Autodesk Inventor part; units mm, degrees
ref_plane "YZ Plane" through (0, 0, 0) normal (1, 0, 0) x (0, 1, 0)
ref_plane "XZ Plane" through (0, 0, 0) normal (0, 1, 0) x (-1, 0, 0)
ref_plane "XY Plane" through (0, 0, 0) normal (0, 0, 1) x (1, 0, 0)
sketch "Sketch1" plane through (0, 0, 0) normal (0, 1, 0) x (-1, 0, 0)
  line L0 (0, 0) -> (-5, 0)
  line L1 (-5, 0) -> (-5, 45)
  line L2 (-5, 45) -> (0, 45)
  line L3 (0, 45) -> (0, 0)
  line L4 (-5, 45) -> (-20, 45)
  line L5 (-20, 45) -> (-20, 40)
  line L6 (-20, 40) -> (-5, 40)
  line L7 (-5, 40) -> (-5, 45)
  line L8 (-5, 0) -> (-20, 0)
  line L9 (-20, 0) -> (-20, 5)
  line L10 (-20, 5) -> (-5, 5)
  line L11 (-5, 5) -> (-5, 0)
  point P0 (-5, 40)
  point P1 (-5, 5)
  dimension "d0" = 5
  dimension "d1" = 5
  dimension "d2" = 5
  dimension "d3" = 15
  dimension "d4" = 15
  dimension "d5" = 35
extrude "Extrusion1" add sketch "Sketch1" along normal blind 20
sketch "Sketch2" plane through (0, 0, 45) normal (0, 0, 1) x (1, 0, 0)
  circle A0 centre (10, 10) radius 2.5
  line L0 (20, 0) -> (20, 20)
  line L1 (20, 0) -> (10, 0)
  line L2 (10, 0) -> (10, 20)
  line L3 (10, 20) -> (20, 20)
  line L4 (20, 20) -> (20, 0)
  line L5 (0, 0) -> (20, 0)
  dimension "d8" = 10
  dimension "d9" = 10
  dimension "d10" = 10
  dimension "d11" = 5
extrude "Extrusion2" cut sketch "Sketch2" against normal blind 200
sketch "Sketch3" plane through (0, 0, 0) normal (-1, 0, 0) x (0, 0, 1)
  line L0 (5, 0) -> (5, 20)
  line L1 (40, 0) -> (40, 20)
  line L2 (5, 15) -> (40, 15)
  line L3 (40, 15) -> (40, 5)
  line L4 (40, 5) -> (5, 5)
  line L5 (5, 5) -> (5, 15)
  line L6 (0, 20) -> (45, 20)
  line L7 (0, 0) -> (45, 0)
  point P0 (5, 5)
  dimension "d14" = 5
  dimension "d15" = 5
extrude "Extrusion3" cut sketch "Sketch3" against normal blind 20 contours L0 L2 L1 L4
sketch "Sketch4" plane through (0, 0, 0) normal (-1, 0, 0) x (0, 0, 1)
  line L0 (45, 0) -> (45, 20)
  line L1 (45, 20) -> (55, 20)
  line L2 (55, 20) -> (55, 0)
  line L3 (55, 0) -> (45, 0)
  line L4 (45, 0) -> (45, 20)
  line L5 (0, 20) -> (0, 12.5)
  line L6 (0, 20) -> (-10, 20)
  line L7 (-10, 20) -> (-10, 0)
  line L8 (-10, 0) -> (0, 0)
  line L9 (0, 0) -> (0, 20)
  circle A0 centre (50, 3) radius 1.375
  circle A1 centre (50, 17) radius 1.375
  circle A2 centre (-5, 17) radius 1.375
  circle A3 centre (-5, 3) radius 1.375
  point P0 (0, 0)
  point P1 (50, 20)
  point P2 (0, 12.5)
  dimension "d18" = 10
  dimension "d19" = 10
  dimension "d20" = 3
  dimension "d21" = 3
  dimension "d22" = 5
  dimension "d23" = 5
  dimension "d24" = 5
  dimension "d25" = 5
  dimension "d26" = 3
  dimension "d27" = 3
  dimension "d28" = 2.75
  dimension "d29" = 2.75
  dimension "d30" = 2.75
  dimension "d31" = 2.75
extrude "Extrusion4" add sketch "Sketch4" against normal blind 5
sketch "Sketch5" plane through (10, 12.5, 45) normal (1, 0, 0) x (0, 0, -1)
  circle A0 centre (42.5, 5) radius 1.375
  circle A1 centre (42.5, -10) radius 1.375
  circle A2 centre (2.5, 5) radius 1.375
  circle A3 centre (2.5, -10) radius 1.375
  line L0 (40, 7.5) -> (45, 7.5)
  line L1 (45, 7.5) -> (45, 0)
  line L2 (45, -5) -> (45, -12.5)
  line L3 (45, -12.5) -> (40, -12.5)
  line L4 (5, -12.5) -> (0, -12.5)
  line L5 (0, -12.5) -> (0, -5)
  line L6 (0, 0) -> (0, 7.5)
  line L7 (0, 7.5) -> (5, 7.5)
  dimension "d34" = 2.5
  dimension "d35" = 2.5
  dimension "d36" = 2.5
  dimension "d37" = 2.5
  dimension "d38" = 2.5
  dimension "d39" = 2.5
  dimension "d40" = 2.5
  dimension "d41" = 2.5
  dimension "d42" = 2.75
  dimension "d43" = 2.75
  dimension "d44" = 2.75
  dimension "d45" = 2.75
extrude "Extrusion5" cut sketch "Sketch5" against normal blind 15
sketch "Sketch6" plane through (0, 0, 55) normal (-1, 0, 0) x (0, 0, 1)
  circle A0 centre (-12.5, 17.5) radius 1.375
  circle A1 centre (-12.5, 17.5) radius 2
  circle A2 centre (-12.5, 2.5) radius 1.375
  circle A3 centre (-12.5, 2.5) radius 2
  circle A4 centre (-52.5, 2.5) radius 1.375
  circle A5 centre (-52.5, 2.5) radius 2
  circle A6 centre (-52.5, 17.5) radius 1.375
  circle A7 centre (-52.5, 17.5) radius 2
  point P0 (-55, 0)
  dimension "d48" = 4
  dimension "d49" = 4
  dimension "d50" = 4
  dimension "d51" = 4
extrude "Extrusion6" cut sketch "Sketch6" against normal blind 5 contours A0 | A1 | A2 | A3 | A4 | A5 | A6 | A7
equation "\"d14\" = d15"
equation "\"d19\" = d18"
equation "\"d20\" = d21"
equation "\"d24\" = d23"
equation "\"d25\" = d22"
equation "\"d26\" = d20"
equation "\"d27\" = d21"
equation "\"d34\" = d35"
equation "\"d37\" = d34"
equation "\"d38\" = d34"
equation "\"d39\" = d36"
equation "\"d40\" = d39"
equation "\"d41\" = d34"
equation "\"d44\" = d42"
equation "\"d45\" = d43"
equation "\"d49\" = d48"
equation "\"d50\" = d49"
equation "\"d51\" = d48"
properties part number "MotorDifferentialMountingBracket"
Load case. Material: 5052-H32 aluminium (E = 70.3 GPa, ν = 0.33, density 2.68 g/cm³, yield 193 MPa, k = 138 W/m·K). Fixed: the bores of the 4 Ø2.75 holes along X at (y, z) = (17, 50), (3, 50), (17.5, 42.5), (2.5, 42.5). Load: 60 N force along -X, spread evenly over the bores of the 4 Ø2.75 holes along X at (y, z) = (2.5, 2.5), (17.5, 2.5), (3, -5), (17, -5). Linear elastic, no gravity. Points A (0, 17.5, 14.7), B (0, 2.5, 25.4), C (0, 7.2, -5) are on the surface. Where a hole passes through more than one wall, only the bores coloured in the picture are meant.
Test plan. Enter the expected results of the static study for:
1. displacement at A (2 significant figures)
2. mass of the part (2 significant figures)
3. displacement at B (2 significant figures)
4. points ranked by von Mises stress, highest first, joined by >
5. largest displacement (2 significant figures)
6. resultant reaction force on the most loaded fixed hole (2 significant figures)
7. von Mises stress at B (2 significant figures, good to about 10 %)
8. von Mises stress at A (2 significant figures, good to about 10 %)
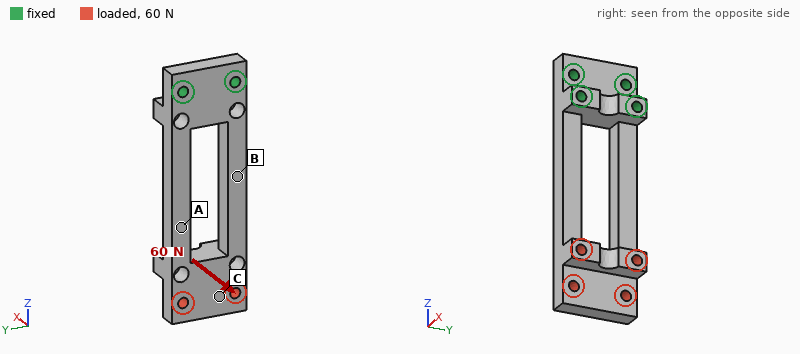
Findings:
0.13 mm
14 g
0.059 mm
B > A > C
0.34 mm
210 N
38 MPa
23 MPa
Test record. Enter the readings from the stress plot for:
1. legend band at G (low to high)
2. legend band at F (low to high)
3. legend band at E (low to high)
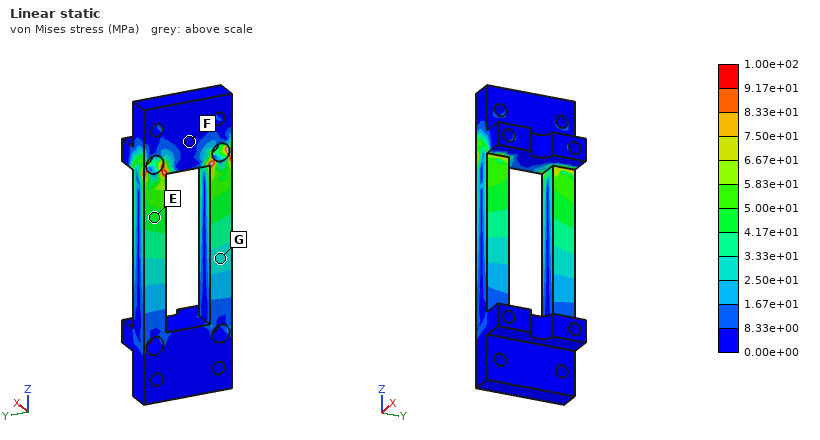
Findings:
2.50e+01 to 3.33e+01 MPa
0.00e+00 to 8.33e+00 MPa
4.17e+01 to 5.00e+01 MPa
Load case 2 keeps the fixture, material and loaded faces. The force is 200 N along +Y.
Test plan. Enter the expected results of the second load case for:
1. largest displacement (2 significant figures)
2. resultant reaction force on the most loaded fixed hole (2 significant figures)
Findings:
0.25 mm
250 N
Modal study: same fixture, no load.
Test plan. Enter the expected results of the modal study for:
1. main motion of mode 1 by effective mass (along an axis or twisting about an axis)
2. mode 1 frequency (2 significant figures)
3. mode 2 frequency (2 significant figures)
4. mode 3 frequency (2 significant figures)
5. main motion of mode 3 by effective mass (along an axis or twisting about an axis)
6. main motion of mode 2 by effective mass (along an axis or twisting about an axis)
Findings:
along X
1000 Hz
2000 Hz
4200 Hz
twisting about Z
along Y
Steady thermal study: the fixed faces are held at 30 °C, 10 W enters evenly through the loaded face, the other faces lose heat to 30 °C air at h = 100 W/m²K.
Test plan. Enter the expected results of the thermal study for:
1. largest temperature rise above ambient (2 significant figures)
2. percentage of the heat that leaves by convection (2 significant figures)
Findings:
33 K
59 %
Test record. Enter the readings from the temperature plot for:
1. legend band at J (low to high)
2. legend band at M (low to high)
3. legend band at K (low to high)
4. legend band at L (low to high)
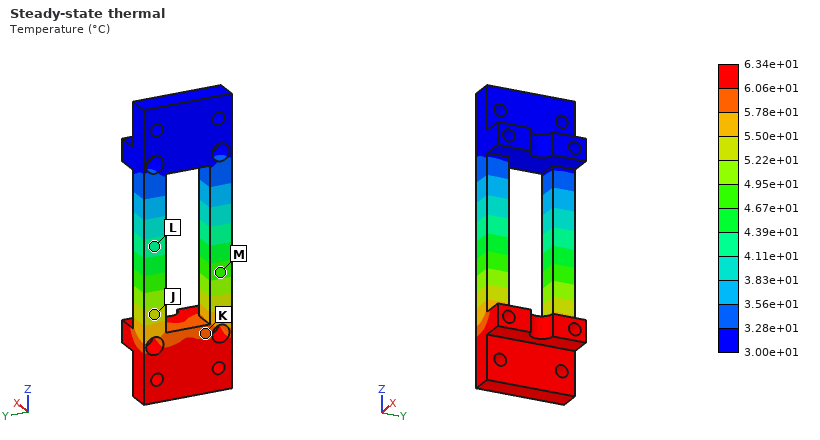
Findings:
5.22e+01 to 5.50e+01 °C
4.67e+01 to 4.95e+01 °C
5.78e+01 to 6.06e+01 °C
4.11e+01 to 4.39e+01 °C
